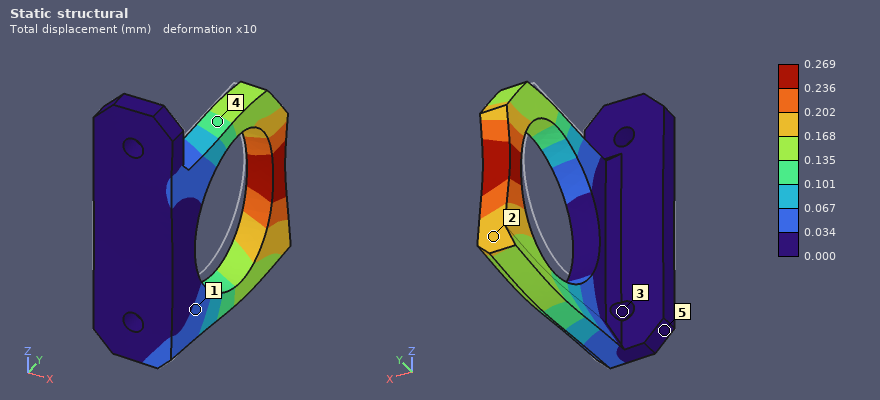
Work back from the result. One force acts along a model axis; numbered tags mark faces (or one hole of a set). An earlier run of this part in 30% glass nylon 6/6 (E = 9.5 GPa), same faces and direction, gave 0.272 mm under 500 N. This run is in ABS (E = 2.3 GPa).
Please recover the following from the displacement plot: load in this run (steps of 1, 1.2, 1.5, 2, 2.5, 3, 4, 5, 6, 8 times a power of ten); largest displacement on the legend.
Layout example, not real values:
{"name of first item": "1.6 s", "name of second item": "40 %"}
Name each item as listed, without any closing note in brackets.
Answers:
{"load in this run": "120 N", "largest displacement on the legend": "0.269 mm"}
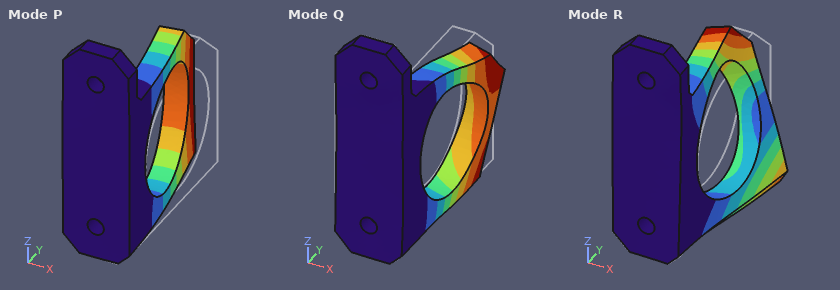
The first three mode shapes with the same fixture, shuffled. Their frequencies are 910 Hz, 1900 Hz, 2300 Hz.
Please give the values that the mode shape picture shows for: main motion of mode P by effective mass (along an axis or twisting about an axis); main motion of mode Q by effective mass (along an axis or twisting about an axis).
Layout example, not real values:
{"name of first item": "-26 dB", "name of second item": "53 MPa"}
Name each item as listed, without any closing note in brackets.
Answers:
{"main motion of mode P by effective mass": "along X", "main motion of mode Q by effective mass": "along Z"}
